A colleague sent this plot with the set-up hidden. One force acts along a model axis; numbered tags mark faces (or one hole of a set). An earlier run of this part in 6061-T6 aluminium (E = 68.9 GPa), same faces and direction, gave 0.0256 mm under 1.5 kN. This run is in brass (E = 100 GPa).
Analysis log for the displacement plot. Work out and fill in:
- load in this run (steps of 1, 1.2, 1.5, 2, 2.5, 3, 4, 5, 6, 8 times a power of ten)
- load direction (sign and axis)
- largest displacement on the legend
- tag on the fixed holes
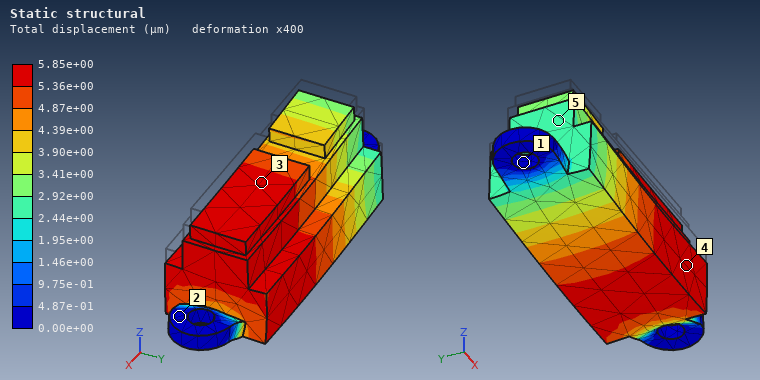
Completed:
500 N
-Z
5.85e+00 µm
1
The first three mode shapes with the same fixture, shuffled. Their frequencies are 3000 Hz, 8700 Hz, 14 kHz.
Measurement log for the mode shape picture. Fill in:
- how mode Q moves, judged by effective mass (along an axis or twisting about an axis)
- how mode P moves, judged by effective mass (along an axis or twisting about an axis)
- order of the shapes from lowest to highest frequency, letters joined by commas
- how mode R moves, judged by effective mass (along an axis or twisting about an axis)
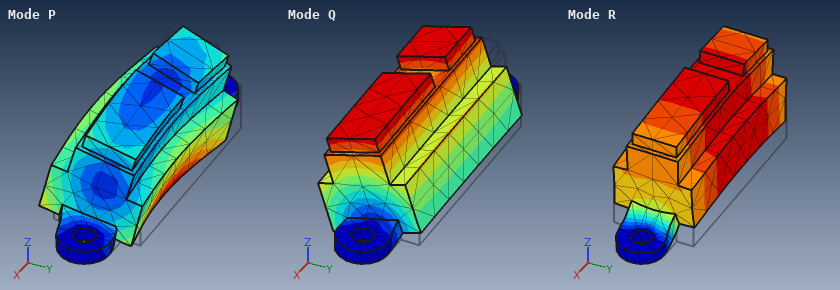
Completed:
along Y
along Y
Q, R, P
along Z
